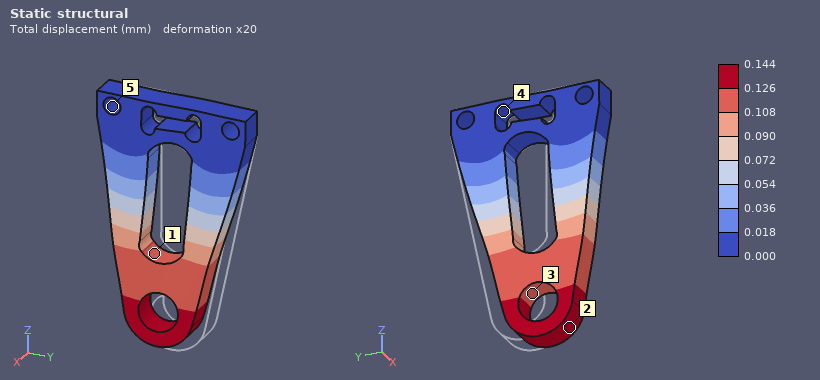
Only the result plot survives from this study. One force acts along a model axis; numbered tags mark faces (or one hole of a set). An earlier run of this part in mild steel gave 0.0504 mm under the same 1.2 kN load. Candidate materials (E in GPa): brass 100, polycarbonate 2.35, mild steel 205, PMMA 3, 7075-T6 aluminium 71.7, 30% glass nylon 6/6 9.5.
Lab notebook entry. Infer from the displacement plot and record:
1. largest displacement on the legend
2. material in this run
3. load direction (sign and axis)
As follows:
0.144 mm
7075-T6 aluminium
-Y
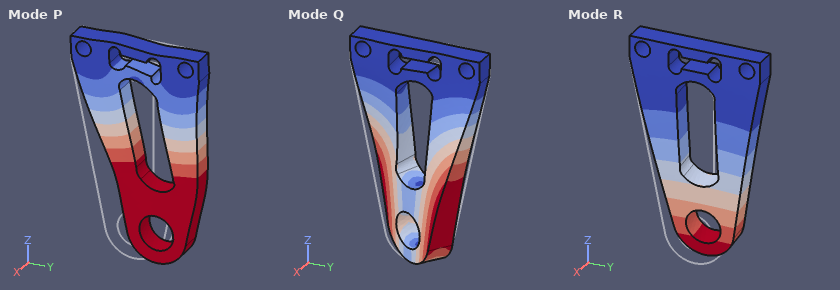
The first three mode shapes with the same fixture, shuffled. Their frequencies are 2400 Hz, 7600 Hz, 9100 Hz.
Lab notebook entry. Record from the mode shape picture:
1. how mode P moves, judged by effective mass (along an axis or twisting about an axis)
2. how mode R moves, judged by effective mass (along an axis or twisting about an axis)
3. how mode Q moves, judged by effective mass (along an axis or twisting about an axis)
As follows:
along Y
along X
twisting about Z
